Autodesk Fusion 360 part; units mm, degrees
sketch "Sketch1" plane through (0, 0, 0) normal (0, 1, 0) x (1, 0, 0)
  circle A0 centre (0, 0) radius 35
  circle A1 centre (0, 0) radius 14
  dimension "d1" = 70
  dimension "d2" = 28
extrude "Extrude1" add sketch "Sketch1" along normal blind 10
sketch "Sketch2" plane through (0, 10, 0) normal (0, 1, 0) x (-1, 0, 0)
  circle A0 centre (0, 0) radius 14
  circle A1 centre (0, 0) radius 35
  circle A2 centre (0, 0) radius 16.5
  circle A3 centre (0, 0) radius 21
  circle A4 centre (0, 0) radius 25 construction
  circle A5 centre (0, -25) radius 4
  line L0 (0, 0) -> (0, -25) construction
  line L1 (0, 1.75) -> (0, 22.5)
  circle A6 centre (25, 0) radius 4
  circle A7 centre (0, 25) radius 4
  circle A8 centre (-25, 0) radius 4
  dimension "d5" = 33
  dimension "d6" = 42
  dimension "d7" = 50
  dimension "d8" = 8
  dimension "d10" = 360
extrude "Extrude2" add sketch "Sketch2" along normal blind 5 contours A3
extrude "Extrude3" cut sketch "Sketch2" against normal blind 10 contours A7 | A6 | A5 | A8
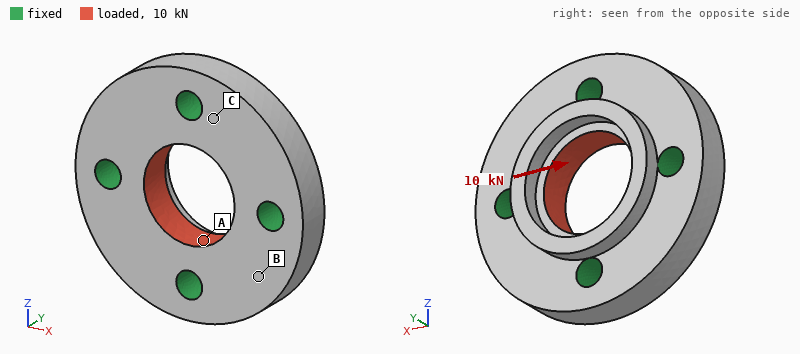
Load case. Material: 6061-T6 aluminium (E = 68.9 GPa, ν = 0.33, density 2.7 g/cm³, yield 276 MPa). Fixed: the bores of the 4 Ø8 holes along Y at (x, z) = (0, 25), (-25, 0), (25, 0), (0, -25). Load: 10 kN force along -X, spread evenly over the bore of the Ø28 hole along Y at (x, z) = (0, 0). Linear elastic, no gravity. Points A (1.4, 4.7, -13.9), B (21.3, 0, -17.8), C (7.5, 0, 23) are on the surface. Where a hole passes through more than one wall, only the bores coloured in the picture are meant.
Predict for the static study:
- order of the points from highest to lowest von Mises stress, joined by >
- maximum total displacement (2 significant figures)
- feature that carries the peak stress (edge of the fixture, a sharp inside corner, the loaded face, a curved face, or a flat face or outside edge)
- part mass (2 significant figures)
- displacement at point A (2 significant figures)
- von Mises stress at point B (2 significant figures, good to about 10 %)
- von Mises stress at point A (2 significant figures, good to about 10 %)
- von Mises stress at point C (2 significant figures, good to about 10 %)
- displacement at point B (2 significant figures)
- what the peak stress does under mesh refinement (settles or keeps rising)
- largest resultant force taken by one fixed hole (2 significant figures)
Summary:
A > C > B
3.7 µm
edge of the fixture
89 g
3.6 µm
4.1 MPa
20 MPa
9.4 MPa
2.1 µm
keeps rising
2.7 kN
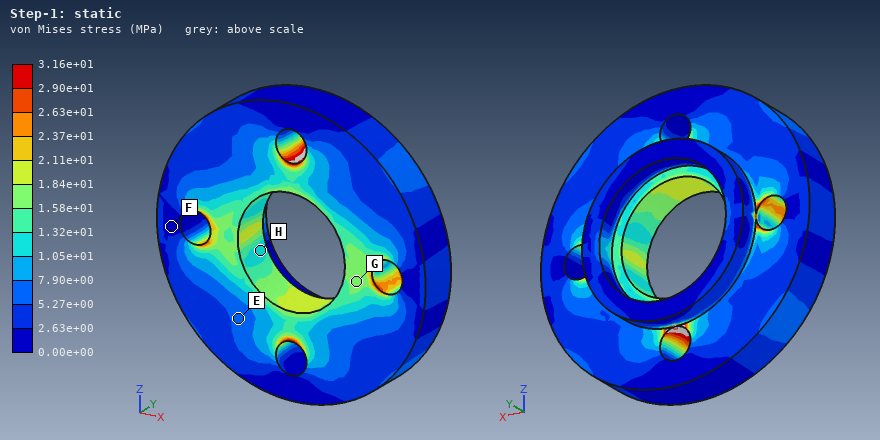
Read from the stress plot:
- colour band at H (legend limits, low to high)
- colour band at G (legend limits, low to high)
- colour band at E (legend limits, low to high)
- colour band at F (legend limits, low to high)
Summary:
1.05e+01 to 1.32e+01 MPa
1.58e+01 to 1.84e+01 MPa
5.27e+00 to 7.90e+00 MPa
0.00e+00 to 2.63e+00 MPa
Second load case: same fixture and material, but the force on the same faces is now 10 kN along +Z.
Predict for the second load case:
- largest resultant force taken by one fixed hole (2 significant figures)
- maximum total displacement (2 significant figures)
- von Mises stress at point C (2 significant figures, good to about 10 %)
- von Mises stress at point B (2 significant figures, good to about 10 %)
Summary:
2.7 kN
3.7 µm
9.6 MPa
4.5 MPa
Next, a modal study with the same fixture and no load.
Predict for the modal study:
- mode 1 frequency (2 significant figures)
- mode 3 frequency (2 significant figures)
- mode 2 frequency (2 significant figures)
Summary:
23 kHz
24 kHz
24 kHz
